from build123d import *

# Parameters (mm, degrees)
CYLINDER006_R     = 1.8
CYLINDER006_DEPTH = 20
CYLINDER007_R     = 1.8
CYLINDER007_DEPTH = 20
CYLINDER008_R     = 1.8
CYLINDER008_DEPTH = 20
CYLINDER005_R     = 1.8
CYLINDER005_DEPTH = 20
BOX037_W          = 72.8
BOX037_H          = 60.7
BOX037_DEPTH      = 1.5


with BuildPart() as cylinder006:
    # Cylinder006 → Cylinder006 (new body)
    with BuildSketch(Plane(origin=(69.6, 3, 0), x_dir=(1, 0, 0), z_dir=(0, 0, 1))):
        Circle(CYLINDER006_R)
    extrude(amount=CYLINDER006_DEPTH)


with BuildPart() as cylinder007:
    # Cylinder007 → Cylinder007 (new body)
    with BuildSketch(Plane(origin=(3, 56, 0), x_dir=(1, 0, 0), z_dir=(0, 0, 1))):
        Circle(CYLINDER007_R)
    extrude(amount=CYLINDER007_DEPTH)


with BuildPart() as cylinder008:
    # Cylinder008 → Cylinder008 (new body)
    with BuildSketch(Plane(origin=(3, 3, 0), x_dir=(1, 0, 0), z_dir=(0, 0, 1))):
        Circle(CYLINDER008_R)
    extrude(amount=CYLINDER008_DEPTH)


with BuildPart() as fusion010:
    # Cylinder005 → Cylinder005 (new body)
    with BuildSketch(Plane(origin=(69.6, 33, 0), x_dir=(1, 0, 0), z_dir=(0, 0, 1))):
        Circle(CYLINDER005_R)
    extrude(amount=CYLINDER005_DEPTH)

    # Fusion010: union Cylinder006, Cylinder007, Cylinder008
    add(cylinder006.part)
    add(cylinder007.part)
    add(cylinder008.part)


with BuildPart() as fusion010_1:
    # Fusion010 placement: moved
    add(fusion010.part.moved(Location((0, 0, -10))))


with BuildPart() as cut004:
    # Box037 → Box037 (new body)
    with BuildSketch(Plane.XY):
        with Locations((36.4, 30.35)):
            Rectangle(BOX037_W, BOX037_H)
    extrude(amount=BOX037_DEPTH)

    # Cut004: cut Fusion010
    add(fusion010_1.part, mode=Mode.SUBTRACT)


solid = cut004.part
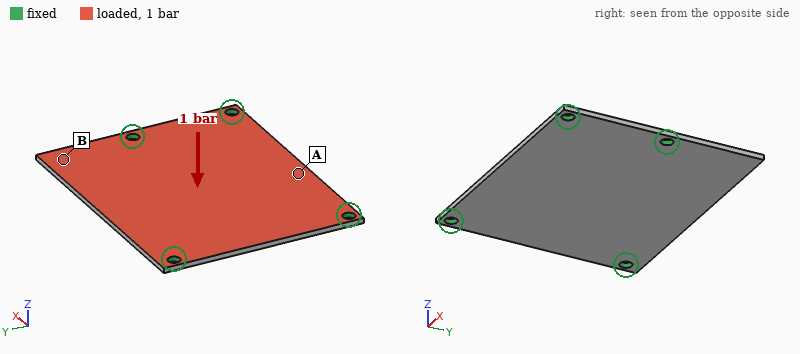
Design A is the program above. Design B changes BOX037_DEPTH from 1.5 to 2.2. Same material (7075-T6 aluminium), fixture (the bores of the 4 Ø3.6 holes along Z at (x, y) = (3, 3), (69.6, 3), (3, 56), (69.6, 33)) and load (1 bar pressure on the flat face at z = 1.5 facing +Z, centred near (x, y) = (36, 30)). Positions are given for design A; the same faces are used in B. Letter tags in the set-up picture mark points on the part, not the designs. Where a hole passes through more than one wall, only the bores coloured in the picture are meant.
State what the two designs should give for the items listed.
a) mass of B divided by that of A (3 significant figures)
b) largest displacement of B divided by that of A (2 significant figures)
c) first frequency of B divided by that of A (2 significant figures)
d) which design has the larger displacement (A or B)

1.47
0.33
1.4
A
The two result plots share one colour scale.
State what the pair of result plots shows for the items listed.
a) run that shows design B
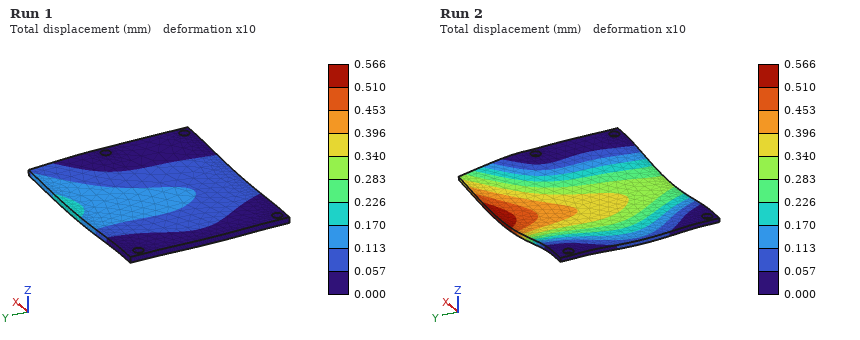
Run 1
